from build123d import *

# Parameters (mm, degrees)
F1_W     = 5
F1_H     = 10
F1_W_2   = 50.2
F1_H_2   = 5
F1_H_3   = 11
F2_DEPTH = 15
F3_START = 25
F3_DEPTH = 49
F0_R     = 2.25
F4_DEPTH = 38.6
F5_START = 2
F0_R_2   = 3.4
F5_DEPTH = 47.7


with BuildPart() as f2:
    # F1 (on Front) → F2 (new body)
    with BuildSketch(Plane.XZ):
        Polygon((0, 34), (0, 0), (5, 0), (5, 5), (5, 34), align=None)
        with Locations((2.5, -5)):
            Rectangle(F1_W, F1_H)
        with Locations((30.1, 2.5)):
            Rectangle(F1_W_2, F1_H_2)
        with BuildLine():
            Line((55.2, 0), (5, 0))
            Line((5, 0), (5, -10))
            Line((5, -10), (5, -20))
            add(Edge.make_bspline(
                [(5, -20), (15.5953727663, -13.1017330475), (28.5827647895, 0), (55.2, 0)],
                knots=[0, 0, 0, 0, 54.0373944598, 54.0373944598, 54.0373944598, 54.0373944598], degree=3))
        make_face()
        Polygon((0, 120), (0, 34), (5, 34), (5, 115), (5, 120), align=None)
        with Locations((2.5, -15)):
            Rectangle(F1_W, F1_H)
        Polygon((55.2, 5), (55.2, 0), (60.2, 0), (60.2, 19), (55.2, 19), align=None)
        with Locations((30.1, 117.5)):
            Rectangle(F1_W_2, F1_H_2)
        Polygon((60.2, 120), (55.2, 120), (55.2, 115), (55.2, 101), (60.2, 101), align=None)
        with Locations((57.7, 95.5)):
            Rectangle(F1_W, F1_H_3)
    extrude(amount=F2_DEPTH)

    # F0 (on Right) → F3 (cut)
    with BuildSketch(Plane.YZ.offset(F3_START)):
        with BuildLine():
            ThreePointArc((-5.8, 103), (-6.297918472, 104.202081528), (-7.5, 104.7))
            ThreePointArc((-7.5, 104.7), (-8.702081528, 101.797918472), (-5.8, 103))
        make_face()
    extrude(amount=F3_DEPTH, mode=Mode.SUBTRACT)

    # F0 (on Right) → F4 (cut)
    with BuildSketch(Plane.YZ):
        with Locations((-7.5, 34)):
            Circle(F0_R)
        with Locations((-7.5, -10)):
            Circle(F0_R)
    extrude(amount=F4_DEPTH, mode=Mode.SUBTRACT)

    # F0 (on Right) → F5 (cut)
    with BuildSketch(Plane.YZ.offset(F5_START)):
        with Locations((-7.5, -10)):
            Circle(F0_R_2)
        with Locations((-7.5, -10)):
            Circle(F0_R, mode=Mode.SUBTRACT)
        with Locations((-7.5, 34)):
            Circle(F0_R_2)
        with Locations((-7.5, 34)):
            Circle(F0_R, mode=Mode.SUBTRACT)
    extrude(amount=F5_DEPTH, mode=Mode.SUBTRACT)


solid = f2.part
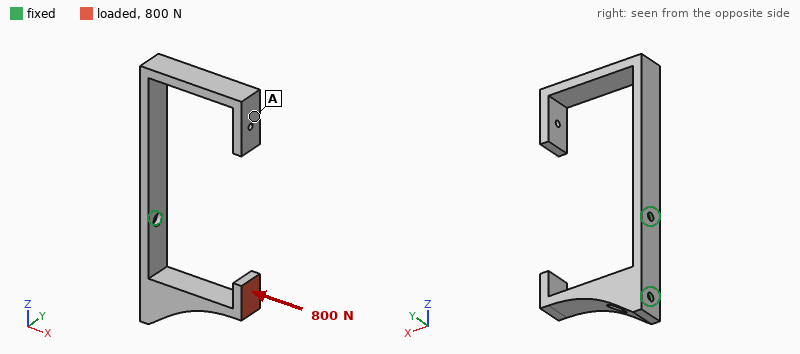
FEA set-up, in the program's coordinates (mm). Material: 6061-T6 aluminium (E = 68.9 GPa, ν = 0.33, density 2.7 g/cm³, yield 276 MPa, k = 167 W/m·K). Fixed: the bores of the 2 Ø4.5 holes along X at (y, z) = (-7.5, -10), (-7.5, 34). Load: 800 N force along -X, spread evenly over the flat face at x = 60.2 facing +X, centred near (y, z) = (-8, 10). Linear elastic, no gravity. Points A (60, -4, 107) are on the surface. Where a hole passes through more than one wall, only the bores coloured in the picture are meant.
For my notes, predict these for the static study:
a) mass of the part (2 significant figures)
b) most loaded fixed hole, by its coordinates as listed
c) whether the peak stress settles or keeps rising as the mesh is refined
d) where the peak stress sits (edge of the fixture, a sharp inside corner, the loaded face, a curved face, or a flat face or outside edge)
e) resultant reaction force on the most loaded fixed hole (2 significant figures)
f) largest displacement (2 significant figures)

70 g
(-7.5, -10)
keeps rising
edge of the fixture
920 N
0.43 mm
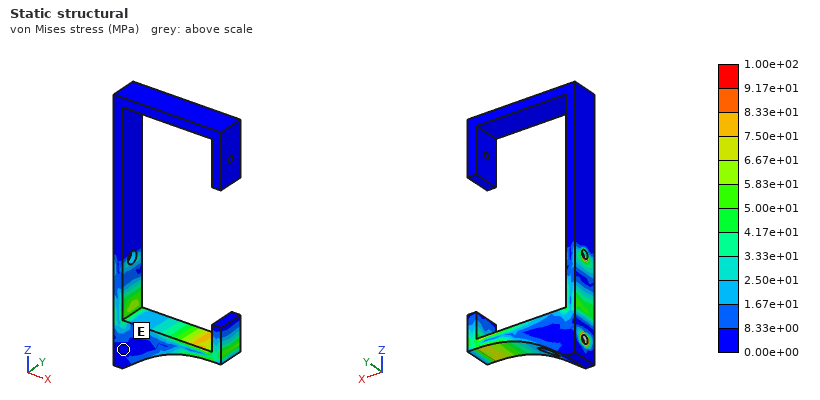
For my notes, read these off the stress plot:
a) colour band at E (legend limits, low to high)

0.00e+00 to 8.33e+00 MPa
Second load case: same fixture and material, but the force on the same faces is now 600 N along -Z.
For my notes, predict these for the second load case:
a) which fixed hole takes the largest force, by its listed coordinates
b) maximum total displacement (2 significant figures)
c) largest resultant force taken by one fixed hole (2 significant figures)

(-7.5, 34)
0.83 mm
1.9 kN
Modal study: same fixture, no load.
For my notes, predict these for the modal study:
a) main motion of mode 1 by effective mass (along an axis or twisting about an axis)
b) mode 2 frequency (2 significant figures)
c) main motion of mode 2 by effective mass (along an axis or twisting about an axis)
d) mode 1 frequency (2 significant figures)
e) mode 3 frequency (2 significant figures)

along X
340 Hz
along Y
210 Hz
560 Hz
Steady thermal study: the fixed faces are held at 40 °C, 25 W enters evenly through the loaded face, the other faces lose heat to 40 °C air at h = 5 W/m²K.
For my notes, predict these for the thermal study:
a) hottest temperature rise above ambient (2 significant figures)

85 K
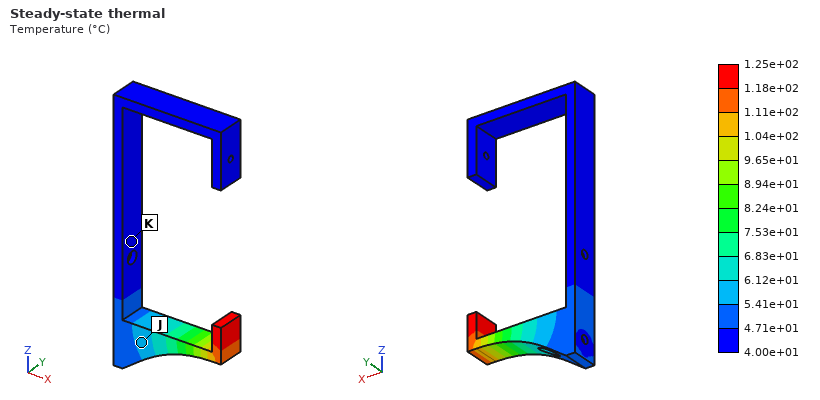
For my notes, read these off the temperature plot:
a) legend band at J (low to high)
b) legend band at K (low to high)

5.41e+01 to 6.12e+01 °C
4.00e+01 to 4.71e+01 °C
